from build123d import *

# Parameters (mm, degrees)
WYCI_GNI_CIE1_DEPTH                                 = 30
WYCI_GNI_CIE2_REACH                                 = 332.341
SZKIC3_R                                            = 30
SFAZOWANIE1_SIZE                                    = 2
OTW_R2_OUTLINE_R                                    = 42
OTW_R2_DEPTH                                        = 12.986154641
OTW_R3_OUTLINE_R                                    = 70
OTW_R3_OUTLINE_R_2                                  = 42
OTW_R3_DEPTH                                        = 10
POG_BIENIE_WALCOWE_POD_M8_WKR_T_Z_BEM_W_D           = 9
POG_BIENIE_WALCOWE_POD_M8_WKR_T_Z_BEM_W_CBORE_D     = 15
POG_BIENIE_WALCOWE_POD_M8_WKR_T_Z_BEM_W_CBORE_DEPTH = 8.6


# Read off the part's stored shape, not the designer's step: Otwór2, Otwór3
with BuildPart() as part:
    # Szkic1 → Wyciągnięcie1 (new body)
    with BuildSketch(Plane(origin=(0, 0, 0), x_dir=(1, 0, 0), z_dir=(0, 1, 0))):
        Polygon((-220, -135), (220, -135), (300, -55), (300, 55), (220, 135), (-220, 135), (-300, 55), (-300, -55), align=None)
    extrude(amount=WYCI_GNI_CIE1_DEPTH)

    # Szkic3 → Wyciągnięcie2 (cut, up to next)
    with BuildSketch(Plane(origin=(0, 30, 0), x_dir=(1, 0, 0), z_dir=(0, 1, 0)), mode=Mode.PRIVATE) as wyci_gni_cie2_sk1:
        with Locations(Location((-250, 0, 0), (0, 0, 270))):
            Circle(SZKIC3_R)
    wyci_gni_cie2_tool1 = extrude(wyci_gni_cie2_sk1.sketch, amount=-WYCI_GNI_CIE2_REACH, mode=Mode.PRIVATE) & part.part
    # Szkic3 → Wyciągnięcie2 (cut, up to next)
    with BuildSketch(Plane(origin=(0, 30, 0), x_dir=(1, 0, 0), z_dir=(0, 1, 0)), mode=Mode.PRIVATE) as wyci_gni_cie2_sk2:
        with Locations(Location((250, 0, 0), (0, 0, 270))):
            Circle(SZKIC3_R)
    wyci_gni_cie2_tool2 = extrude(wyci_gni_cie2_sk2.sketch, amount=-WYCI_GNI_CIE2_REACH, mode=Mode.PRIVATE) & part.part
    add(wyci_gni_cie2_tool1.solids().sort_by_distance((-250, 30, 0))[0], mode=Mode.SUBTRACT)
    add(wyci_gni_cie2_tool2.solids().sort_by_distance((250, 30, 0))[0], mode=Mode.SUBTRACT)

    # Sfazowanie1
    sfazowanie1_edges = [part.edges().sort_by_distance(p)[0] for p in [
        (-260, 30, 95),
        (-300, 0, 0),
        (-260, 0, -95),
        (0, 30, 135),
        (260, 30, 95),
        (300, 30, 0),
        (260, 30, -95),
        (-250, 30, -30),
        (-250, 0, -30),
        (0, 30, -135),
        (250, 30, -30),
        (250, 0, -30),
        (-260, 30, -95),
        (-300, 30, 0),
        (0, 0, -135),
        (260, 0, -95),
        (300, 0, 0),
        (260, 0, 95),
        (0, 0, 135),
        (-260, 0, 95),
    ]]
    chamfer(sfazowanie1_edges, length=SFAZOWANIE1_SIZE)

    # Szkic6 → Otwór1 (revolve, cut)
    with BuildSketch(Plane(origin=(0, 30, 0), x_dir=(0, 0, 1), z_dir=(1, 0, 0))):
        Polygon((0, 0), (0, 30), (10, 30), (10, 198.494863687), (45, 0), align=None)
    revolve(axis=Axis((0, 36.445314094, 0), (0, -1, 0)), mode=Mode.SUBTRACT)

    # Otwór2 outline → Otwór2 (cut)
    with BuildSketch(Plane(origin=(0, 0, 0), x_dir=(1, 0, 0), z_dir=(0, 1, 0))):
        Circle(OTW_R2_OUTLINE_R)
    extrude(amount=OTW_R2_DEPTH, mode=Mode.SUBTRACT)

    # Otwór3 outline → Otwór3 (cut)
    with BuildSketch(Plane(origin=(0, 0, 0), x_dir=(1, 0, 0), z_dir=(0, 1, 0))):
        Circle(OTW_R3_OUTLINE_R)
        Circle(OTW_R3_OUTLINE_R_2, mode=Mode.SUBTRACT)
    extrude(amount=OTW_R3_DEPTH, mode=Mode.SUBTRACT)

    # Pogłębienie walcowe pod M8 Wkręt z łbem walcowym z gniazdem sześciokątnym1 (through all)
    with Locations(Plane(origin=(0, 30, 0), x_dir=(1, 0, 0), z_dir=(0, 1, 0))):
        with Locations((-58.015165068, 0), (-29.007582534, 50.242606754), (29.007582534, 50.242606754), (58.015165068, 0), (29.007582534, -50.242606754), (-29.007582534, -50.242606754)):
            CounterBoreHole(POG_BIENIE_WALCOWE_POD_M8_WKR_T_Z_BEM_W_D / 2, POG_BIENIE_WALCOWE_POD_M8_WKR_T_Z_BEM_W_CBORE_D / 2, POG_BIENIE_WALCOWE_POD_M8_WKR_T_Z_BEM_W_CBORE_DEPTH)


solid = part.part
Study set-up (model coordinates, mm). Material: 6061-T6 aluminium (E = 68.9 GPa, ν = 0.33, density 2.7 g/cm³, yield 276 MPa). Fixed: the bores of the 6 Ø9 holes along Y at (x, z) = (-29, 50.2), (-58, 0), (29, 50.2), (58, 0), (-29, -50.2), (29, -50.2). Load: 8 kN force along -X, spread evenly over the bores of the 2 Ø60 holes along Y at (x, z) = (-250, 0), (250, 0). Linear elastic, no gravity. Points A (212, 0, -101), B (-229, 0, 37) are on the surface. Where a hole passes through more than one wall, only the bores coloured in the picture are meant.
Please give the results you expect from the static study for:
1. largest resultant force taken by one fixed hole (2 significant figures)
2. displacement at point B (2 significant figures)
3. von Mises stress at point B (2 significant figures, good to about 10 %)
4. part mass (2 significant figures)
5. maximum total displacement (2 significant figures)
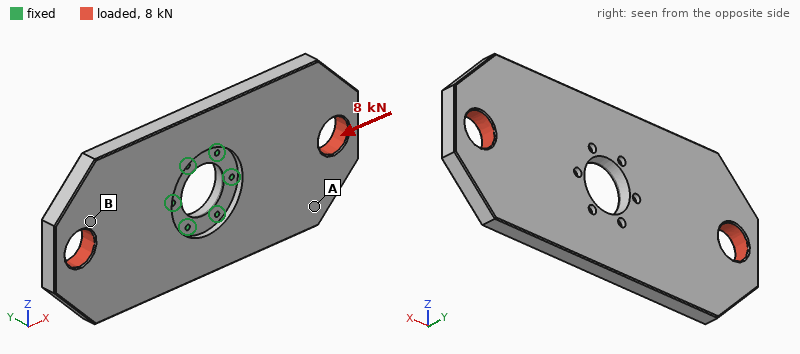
1.3 kN
4.9 µm
1.2 MPa
11 kg
7.2 µm
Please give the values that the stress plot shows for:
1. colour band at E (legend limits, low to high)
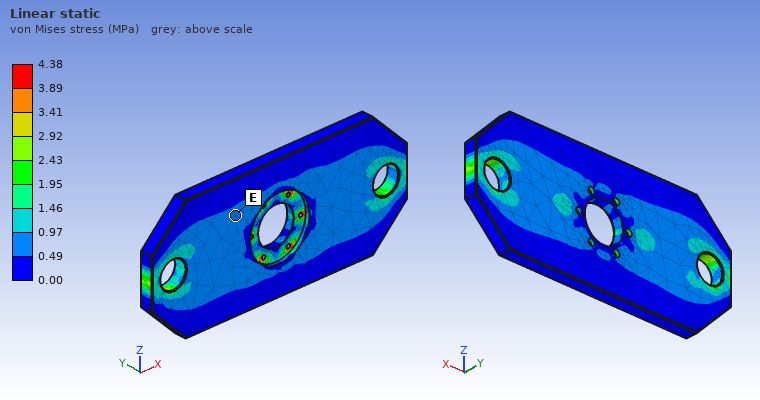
0.49 to 0.97 MPa
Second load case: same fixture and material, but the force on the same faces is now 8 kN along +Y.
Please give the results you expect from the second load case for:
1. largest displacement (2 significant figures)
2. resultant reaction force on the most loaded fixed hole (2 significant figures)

0.69 mm
7.7 kN
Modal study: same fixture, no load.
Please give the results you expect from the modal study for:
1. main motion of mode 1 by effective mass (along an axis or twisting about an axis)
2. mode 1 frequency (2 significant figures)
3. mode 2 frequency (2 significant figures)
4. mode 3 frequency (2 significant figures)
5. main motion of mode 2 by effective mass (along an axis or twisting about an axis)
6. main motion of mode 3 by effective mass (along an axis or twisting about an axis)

twisting about Z
300 Hz
330 Hz
650 Hz
along Y
twisting about X
